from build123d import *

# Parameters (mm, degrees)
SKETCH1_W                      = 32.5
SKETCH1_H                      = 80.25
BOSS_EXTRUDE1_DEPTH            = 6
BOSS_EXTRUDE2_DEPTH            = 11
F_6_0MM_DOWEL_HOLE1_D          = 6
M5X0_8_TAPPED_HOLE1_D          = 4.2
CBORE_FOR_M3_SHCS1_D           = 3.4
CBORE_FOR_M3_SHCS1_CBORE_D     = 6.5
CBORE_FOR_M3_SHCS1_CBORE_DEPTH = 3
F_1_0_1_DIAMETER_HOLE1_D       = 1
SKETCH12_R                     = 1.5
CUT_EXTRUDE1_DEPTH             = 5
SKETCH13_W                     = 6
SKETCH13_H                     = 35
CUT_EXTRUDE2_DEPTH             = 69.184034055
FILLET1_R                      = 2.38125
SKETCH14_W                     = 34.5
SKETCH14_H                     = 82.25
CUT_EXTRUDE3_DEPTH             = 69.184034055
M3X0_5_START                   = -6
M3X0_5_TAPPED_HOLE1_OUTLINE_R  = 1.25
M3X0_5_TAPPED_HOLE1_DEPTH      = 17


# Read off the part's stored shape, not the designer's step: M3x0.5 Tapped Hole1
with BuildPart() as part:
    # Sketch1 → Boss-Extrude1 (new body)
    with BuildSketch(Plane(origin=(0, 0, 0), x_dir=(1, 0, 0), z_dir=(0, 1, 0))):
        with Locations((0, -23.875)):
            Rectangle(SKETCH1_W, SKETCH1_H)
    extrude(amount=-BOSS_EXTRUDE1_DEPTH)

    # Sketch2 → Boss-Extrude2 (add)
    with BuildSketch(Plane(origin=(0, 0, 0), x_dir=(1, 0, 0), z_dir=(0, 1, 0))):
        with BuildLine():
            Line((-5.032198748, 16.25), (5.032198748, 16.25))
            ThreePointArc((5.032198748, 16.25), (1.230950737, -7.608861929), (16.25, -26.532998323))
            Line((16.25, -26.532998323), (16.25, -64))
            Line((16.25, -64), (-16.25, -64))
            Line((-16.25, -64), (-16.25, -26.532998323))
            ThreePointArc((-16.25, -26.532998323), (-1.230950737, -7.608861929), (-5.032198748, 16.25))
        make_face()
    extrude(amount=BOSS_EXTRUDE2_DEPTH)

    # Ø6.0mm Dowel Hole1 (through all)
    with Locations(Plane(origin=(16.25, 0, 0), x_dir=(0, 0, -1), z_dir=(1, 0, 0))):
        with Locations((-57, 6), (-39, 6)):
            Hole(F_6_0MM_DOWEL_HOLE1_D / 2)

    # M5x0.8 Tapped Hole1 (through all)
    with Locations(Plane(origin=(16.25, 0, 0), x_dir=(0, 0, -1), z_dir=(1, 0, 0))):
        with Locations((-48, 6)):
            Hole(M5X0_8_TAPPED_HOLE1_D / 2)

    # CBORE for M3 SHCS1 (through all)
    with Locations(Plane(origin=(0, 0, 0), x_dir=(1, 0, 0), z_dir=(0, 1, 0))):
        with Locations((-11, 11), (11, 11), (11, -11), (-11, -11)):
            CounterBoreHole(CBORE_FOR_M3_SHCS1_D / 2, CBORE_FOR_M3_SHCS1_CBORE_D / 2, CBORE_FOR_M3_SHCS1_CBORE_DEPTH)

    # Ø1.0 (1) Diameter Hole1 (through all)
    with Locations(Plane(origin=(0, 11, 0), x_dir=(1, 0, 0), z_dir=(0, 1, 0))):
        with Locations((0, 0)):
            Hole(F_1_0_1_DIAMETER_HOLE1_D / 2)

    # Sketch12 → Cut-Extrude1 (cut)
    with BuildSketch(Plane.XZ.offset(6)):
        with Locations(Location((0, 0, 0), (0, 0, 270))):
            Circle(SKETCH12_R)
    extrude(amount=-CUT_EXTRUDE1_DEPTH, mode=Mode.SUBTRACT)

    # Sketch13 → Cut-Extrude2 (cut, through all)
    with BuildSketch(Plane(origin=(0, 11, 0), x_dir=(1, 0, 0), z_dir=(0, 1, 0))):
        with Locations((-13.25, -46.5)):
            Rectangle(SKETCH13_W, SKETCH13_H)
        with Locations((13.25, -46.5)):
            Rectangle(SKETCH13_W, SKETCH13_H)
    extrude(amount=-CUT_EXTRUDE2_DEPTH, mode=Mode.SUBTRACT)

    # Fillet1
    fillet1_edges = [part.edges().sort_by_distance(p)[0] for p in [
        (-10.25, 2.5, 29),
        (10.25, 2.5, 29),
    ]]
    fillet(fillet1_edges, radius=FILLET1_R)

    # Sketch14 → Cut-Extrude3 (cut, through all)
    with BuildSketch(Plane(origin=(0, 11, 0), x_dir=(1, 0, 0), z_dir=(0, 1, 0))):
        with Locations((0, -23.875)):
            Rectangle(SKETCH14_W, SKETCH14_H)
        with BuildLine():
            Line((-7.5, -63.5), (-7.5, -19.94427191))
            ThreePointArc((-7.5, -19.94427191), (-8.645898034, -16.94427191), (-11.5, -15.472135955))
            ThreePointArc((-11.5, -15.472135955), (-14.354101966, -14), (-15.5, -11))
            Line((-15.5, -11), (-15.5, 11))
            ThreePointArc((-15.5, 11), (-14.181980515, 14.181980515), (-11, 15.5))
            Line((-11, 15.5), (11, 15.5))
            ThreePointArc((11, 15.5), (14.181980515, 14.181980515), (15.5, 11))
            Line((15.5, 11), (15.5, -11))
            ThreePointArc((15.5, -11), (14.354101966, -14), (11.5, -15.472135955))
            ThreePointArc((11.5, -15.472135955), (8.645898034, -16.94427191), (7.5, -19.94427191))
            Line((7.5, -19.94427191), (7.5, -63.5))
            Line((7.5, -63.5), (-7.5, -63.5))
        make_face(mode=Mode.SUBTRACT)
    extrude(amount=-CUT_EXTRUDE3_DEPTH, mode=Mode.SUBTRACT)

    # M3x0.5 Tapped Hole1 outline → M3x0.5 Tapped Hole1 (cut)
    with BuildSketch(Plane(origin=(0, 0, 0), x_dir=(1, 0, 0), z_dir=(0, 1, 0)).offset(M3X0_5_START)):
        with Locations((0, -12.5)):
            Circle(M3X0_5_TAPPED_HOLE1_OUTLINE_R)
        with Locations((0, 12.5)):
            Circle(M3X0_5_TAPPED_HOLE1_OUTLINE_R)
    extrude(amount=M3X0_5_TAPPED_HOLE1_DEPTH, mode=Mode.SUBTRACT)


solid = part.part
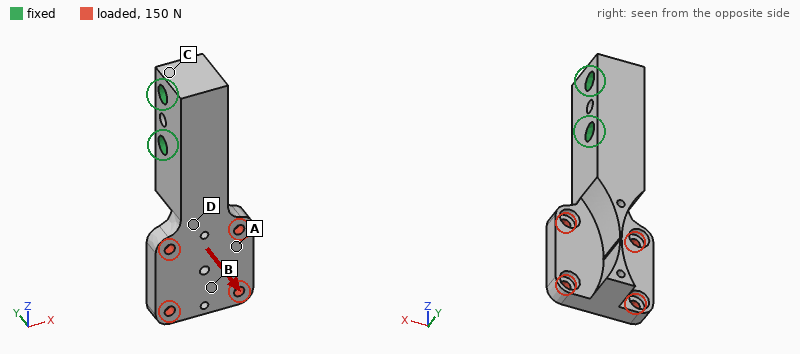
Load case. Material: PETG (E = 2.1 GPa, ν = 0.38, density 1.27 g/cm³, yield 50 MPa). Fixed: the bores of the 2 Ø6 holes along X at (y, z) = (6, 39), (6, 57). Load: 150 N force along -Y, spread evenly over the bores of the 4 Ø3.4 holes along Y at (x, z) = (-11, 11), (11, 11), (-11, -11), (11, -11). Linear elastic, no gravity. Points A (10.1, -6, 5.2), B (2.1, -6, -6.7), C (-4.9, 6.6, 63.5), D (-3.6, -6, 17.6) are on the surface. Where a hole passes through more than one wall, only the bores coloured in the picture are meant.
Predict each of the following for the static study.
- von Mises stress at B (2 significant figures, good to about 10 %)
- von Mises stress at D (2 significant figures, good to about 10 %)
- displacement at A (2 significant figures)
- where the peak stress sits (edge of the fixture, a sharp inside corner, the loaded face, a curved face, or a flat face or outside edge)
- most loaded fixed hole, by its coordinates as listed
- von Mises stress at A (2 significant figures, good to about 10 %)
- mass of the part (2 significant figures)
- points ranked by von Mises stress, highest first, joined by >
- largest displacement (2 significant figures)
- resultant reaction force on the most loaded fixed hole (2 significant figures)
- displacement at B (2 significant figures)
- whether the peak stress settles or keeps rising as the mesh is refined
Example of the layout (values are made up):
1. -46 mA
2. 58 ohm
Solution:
1. 2.3 MPa
2. 5.7 MPa
3. 0.36 mm
4. a sharp inside corner
5. (6, 39)
6. 4.2 MPa
7. 22 g
8. D > A > B > C
9. 0.90 mm
10. 340 N
11. 0.63 mm
12. keeps rising
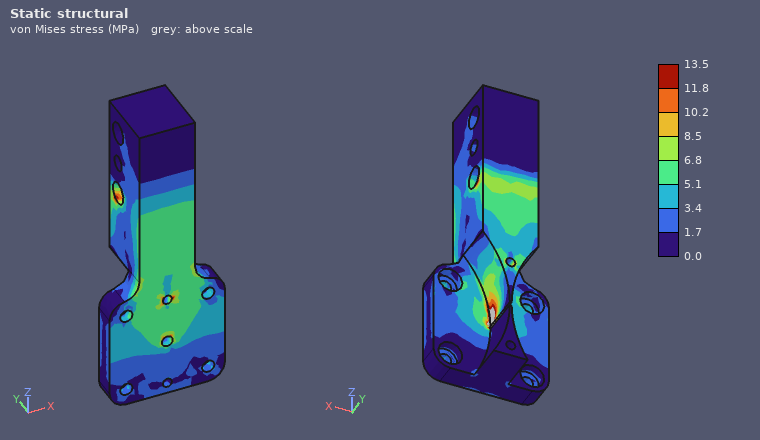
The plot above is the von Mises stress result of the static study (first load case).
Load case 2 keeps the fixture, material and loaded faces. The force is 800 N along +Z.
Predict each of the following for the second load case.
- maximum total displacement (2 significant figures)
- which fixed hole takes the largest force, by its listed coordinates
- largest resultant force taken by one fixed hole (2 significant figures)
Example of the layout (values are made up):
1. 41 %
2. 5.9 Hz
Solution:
1. 0.94 mm
2. (6, 39)
3. 550 N
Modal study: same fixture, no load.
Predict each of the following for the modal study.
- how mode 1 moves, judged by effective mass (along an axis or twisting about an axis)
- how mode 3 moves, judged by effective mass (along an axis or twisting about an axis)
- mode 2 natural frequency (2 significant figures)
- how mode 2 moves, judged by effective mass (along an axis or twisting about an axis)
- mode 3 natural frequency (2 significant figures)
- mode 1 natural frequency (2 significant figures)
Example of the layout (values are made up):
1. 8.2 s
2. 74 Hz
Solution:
1. along Y
2. twisting about Z
3. 1000 Hz
4. along X
5. 1700 Hz
6. 920 Hz
